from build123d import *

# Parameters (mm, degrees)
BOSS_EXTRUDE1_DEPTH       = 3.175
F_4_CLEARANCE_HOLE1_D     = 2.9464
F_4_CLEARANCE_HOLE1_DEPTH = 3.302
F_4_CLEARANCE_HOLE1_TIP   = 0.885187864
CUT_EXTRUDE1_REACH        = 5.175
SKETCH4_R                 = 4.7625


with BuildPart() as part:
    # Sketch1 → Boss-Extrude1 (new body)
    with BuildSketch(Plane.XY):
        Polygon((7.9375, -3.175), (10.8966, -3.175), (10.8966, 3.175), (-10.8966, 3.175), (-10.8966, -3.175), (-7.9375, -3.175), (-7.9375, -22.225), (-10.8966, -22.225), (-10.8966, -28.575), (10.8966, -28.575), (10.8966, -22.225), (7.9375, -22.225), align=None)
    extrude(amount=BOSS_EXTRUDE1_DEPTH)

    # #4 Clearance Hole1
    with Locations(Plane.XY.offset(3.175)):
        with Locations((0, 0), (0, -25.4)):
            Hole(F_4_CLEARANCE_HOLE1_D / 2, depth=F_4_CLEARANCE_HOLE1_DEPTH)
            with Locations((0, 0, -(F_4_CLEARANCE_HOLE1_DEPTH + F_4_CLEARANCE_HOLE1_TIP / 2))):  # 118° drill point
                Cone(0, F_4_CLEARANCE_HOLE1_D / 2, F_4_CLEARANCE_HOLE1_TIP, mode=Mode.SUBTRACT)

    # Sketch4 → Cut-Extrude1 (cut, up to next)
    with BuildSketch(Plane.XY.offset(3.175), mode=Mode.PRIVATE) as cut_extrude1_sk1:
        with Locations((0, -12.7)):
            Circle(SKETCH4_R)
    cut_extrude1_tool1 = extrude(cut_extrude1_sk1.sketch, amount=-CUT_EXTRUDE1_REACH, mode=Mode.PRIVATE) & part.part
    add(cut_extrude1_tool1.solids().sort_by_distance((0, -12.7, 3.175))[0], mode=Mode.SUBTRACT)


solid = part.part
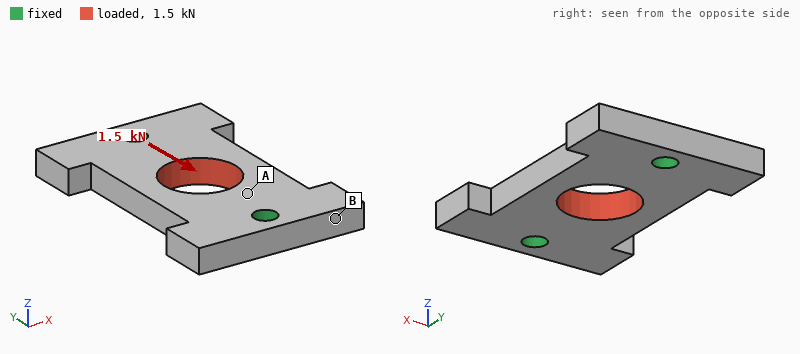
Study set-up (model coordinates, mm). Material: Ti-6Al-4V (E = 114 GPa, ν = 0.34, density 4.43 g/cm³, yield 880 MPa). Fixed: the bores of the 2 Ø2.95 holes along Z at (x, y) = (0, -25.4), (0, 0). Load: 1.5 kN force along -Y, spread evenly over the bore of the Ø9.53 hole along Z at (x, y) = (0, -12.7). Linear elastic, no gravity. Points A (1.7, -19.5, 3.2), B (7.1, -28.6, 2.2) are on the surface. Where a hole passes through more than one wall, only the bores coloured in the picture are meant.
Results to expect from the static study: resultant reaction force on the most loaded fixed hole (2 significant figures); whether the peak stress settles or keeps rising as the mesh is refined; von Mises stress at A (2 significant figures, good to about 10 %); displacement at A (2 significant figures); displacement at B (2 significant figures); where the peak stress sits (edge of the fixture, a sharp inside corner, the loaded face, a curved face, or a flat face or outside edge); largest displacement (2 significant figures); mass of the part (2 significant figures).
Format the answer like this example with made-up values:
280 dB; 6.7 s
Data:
750 N; keeps rising; 26 MPa; 1.3 µm; 1.6 µm; edge of the fixture; 2.8 µm; 7.0 g
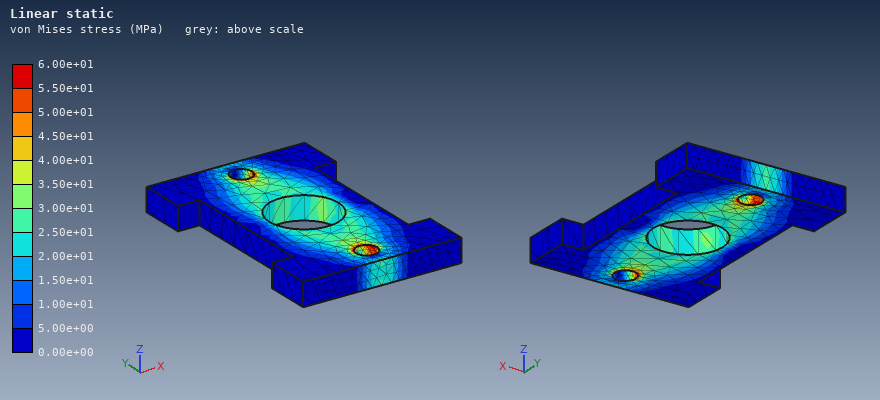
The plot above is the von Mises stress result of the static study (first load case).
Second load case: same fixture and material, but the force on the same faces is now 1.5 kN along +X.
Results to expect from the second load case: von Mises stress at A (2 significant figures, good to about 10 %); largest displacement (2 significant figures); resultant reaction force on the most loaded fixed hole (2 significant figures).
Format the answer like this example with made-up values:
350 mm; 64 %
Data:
37 MPa; 7.9 µm; 750 N
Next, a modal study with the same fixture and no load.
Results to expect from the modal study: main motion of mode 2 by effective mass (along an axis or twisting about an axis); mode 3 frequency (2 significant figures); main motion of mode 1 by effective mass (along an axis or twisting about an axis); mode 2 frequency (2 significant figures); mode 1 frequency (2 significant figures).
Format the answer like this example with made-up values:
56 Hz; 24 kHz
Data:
along Z; 26 kHz; twisting about Y; 22 kHz; 19 kHz
